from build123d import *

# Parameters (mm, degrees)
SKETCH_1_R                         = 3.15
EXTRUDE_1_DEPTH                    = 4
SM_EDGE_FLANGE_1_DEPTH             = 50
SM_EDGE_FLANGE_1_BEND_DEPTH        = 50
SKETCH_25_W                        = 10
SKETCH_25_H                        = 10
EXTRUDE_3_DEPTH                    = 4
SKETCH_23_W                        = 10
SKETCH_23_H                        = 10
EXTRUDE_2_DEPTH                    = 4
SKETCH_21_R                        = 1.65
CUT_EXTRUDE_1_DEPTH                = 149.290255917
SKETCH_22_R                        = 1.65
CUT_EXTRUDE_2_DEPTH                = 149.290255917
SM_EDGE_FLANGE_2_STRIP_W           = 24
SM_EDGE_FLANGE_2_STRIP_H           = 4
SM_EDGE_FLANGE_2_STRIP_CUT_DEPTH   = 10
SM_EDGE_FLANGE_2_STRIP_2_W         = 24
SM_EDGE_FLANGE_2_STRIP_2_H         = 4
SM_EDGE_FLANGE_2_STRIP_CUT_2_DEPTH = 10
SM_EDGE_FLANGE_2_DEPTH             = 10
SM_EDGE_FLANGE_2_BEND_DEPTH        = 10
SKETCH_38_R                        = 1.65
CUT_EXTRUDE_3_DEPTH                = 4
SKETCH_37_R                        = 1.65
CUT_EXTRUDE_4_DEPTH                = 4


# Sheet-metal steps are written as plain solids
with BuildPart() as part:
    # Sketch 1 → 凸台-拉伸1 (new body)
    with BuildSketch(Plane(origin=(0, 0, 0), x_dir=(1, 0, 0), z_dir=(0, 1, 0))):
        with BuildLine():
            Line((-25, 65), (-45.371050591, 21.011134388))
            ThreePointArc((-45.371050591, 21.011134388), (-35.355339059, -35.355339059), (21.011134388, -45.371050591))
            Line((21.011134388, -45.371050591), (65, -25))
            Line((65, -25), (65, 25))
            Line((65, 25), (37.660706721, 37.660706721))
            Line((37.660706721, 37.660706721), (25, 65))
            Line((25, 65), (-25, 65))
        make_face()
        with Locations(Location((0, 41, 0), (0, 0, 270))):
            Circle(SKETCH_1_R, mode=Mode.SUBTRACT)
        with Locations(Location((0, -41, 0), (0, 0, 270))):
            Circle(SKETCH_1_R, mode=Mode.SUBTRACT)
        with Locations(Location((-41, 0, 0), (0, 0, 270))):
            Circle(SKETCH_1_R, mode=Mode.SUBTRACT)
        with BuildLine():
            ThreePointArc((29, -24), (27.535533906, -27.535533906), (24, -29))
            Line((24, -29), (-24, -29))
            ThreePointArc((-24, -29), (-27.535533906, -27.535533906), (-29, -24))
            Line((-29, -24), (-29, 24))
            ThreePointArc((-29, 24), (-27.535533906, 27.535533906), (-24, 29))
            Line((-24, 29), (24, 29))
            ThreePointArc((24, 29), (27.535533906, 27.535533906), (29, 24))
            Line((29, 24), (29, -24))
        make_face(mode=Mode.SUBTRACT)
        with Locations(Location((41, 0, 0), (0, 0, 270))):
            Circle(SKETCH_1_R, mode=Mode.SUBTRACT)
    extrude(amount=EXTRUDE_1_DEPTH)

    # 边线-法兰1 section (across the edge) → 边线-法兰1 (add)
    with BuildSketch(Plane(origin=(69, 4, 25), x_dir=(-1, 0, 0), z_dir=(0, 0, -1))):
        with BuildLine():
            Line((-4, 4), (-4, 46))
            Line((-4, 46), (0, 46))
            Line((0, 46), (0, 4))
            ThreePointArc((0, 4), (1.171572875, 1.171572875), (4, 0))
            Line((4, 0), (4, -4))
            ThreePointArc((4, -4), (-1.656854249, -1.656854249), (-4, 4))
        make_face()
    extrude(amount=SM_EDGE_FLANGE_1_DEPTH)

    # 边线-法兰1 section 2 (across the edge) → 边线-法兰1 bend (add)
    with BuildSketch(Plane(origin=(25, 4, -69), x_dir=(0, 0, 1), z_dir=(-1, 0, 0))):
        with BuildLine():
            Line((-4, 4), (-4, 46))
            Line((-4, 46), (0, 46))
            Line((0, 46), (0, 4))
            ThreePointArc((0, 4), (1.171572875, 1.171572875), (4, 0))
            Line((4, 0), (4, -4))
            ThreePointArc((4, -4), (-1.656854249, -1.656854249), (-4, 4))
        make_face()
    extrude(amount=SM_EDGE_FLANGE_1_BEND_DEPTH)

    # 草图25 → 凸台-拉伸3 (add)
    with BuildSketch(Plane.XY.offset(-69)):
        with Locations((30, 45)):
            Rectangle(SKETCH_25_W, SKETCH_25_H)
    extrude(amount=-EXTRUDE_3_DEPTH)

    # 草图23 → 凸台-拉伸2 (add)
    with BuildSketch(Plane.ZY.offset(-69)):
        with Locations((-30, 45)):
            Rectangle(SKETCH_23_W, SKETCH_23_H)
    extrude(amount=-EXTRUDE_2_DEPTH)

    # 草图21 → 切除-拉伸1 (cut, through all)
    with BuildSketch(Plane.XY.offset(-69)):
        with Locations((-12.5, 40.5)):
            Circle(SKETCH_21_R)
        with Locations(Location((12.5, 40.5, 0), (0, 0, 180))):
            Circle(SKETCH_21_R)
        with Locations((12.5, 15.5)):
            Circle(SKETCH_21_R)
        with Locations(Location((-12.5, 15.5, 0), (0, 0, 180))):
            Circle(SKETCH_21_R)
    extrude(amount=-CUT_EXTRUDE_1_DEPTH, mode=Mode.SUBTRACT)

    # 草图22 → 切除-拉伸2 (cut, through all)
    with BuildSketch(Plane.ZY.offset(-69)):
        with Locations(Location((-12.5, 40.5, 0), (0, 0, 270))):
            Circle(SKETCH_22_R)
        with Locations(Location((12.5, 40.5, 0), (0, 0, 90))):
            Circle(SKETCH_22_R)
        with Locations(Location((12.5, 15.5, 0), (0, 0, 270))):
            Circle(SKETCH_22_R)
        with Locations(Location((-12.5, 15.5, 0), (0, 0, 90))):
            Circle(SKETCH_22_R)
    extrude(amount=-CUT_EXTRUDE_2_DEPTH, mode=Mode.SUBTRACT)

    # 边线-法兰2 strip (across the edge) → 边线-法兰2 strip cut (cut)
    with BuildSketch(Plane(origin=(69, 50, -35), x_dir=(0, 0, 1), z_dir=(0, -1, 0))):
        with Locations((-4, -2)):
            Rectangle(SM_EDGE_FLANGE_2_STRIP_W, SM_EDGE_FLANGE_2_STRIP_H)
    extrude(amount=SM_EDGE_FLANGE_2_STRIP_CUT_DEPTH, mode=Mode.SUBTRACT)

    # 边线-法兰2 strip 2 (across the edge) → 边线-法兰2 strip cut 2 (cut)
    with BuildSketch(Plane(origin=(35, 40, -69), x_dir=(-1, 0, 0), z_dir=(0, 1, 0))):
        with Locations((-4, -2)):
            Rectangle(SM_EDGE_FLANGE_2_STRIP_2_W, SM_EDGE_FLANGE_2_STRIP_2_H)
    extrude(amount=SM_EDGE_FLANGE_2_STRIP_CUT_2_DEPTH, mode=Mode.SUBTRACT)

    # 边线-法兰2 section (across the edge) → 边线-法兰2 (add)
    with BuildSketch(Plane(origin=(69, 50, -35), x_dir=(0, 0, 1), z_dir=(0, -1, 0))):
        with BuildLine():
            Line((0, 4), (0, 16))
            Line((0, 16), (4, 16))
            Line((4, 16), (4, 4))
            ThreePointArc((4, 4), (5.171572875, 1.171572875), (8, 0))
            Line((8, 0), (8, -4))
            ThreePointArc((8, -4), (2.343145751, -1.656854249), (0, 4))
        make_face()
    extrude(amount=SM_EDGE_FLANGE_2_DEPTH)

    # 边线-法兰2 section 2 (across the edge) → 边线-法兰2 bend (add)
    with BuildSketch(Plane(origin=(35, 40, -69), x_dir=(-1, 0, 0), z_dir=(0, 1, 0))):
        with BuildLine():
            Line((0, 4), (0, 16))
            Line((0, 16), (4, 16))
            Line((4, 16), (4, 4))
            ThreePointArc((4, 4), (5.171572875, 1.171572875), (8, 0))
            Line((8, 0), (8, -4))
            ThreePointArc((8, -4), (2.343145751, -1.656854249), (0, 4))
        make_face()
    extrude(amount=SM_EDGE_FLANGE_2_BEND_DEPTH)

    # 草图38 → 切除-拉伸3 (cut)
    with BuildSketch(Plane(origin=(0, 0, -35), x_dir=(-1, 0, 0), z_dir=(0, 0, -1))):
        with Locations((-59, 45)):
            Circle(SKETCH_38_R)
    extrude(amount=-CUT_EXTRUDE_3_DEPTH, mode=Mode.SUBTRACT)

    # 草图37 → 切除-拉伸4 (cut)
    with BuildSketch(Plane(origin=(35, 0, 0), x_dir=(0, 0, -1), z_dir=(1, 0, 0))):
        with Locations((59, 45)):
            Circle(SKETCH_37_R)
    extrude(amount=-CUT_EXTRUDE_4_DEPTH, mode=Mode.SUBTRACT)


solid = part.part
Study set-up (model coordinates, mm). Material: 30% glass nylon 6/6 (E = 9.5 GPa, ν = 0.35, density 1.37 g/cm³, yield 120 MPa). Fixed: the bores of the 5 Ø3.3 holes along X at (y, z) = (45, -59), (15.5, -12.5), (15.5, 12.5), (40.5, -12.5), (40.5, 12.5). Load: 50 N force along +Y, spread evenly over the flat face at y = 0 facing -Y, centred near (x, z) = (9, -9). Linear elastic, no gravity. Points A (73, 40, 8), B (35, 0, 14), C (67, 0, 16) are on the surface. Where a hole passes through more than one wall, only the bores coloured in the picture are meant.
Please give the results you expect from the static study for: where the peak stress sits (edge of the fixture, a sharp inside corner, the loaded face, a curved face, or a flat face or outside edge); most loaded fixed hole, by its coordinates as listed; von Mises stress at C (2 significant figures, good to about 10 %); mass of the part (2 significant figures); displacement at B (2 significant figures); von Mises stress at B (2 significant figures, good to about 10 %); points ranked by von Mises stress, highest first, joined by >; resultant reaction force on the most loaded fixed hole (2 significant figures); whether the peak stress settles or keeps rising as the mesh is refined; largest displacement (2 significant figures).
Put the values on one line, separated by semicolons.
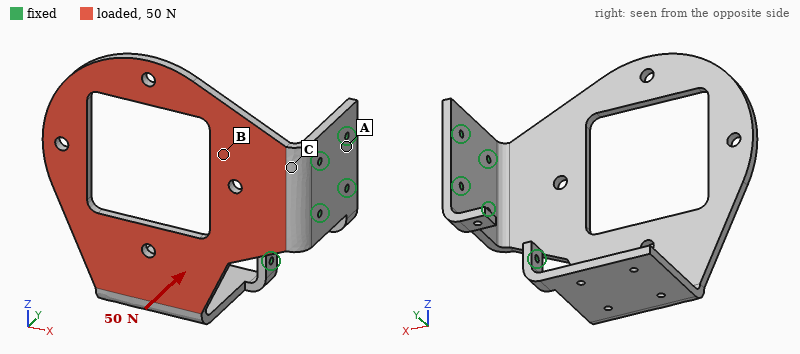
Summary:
edge of the fixture; (15.5, -12.5); 8.0 MPa; 67 g; 0.38 mm; 5.1 MPa; C > B > A; 93 N; keeps rising; 2.0 mm
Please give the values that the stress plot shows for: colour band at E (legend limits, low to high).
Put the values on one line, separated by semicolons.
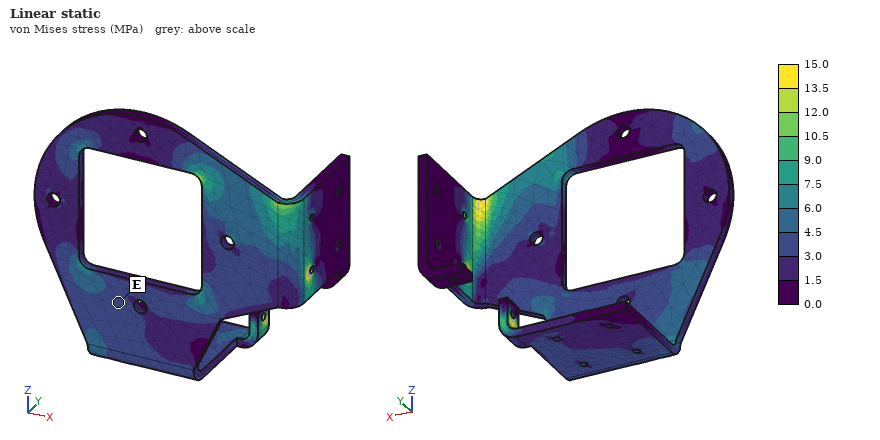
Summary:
3.0 to 4.5 MPa
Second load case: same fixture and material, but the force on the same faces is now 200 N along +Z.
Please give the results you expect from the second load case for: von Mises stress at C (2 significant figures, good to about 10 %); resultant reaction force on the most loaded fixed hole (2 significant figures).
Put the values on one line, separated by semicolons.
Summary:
15 MPa; 390 N
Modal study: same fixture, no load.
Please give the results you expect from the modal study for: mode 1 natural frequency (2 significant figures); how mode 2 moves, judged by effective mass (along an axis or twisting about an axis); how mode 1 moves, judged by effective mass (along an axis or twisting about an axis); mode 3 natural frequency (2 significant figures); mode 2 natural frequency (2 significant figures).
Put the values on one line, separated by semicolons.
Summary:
170 Hz; along Z; along Y; 520 Hz; 280 Hz
